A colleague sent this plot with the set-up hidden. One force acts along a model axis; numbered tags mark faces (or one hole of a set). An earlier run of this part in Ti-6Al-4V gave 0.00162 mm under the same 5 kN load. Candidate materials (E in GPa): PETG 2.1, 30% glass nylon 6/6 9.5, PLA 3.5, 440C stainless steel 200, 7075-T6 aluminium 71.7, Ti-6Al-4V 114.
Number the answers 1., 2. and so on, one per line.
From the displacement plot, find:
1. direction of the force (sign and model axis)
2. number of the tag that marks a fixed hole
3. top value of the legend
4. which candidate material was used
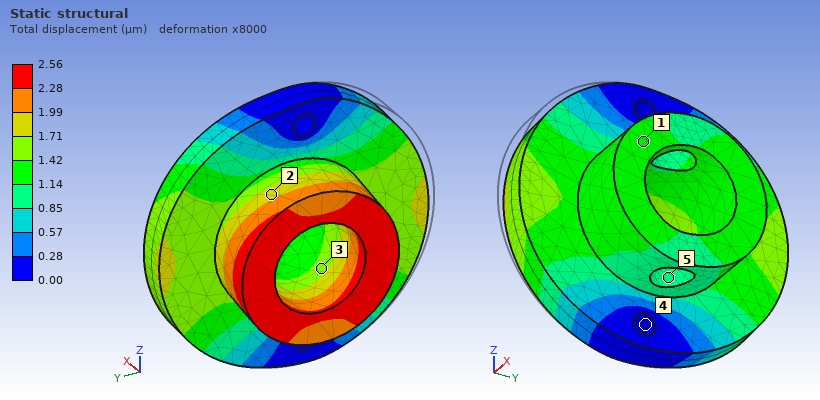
1. +Y
2. 4
3. 2.56 µm
4. 7075-T6 aluminium
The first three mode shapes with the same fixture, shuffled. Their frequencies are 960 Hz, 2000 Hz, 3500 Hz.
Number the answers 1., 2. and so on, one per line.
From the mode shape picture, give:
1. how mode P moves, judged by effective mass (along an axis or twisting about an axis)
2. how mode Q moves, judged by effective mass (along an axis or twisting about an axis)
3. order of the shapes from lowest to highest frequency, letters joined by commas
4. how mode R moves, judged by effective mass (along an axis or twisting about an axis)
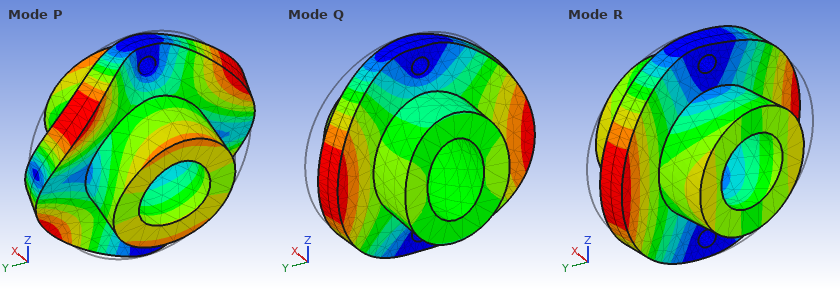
1. twisting about Y
2. along X
3. R, Q, P
4. twisting about Z
